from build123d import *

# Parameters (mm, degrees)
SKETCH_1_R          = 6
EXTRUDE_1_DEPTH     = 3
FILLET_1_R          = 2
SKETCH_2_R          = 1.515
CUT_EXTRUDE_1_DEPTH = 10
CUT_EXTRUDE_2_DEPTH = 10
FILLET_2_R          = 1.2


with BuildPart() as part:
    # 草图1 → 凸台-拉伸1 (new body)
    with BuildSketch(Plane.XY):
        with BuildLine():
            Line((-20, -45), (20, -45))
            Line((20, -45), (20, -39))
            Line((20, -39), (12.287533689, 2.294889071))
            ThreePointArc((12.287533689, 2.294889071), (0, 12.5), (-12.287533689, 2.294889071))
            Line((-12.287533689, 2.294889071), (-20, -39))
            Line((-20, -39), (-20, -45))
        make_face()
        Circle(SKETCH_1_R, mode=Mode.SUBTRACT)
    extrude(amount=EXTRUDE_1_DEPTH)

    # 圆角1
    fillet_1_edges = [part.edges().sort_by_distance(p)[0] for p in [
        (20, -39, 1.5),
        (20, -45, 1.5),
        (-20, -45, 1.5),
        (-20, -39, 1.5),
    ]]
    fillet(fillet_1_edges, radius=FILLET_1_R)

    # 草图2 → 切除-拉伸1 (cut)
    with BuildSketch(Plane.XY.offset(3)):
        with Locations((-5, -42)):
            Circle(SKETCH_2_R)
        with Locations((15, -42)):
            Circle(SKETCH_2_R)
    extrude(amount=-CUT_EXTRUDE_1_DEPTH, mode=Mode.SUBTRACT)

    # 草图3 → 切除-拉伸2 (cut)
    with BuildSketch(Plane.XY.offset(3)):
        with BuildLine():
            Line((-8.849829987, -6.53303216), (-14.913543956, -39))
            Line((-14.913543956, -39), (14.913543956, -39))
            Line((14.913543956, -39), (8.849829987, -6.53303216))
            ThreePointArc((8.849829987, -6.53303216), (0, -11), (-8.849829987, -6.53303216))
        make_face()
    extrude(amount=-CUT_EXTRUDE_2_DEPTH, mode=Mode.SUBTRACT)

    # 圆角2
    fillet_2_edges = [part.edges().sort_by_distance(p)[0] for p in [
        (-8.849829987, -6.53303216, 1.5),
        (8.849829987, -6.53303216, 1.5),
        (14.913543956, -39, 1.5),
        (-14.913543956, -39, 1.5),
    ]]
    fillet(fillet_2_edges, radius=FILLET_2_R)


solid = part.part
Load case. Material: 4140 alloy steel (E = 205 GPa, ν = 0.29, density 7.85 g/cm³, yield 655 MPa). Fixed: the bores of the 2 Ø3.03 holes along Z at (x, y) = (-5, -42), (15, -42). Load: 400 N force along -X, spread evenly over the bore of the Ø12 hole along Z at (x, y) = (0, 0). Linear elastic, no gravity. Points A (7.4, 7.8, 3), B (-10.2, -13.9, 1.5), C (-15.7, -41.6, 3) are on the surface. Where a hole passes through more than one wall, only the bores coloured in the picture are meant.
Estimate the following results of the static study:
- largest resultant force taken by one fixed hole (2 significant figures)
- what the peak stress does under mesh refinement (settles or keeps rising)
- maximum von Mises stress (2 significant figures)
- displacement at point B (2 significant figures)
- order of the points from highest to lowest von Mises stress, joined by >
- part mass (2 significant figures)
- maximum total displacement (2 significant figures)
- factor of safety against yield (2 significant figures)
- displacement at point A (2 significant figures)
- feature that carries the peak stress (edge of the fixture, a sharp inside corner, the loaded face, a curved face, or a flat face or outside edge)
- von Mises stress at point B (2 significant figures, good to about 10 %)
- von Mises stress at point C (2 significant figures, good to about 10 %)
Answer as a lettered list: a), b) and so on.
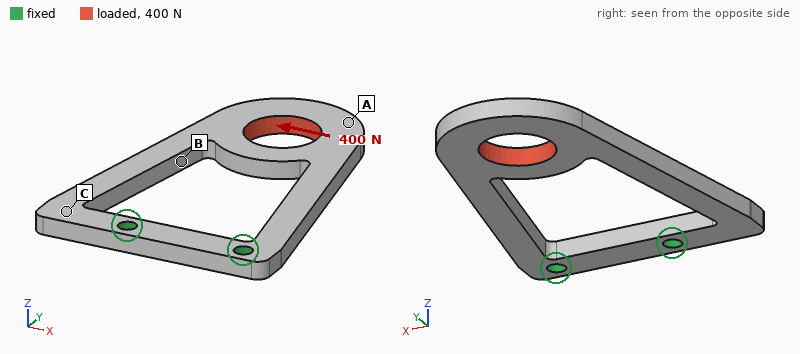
a) 470 N
b) settles
c) 430 MPa
d) 0.12 mm
e) B > C > A
f) 22 g
g) 0.14 mm
h) 1.5
i) 0.14 mm
j) a curved face
k) 140 MPa
l) 69 MPa
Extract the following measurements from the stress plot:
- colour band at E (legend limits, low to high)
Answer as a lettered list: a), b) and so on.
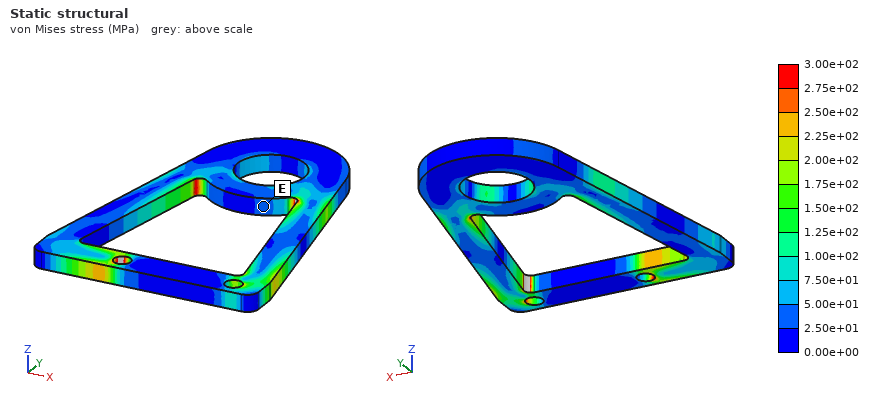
a) 2.50e+01 to 5.00e+01 MPa
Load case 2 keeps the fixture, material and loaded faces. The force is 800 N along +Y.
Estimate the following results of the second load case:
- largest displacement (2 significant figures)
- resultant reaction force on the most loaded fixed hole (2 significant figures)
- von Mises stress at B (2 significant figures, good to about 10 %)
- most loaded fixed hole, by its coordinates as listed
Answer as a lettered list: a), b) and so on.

a) 44 µm
b) 440 N
c) 31 MPa
d) (-5, -42)
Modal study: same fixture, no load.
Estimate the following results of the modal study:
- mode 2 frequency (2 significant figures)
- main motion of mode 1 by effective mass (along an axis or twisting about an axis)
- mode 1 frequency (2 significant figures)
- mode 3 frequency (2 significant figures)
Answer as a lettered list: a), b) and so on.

a) 2500 Hz
b) along Z
c) 620 Hz
d) 2500 Hz
